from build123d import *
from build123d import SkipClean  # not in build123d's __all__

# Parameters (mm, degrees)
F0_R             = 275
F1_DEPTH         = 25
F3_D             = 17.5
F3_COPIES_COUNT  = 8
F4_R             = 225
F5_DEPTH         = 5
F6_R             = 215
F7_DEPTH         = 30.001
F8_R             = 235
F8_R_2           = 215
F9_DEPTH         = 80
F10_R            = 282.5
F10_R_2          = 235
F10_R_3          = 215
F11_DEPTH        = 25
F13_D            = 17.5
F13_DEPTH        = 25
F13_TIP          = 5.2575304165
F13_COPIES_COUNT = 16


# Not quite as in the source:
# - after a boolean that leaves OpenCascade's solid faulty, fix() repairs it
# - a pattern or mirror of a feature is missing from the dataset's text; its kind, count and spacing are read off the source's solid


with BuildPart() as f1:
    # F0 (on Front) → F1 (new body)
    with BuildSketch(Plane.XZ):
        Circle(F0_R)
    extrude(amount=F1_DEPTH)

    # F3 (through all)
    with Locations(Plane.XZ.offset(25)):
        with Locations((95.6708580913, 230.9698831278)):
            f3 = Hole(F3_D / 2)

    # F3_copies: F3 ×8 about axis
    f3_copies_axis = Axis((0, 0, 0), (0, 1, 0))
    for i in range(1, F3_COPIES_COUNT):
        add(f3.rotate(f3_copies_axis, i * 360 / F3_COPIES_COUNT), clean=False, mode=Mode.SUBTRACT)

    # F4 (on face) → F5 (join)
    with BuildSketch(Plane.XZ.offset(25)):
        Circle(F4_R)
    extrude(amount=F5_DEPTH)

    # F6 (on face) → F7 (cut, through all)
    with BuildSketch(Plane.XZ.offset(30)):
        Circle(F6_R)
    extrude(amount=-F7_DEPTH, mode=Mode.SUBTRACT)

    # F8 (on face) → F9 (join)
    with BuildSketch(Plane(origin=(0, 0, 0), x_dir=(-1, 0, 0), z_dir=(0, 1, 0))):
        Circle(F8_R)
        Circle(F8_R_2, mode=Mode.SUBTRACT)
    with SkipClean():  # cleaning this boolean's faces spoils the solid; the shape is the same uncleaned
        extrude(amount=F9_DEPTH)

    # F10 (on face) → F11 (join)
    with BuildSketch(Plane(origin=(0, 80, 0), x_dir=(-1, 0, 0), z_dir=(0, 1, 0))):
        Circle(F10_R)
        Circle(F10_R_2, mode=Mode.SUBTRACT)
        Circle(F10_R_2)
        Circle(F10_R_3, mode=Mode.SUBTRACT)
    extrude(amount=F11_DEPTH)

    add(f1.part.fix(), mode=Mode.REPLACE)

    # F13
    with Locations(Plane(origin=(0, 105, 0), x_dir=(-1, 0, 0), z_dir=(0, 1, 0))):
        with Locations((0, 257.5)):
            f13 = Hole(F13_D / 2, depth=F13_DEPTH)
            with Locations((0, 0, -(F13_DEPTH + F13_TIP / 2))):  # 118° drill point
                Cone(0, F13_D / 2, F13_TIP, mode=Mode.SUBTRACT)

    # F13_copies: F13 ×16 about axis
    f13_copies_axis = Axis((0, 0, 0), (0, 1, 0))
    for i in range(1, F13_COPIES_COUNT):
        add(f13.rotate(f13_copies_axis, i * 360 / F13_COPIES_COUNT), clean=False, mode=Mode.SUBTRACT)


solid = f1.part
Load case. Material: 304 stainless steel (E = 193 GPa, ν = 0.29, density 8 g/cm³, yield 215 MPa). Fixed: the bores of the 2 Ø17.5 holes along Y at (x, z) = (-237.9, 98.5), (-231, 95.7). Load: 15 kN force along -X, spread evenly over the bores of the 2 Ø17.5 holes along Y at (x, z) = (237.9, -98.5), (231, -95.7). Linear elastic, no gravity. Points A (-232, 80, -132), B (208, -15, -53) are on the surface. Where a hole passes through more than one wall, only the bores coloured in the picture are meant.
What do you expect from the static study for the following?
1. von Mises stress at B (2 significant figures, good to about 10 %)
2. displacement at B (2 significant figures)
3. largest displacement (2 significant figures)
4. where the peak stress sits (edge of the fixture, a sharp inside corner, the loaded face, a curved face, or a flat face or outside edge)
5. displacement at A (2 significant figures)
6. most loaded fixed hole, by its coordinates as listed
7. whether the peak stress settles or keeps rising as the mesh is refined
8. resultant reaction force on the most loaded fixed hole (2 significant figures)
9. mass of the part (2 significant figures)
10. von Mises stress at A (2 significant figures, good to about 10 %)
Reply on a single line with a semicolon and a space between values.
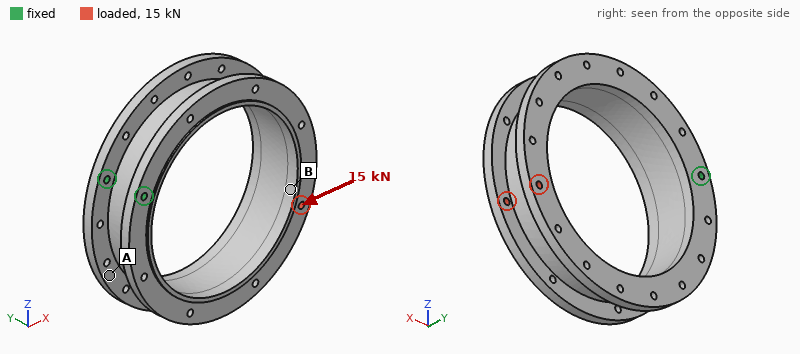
17 MPa; 0.65 mm; 0.74 mm; edge of the fixture; 0.32 mm; (-231, 95.7); keeps rising; 8.3 kN; 57 kg; 8.6 MPa
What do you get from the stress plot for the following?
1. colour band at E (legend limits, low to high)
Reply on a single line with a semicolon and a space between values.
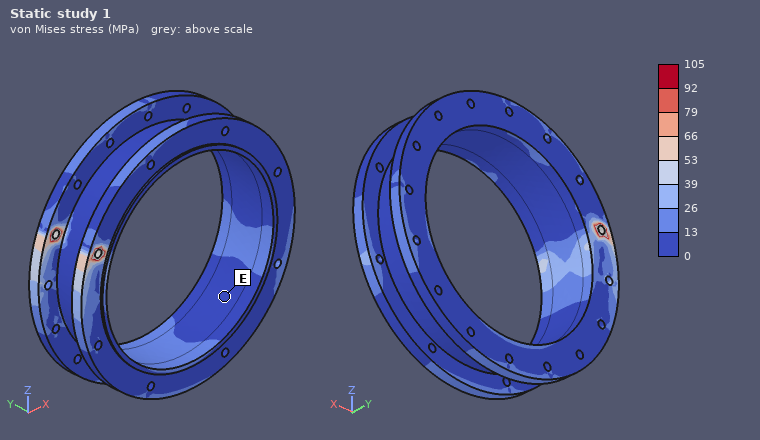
0 to 13 MPa
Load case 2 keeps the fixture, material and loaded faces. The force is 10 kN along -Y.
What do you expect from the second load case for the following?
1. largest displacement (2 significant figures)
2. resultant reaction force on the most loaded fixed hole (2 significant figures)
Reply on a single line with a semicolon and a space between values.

1.6 mm; 43 kN
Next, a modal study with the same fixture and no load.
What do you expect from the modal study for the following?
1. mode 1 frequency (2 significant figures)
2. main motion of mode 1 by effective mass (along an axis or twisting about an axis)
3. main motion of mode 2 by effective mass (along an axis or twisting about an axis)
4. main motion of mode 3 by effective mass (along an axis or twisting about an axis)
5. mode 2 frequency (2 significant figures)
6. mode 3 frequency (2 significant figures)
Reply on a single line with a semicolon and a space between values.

89 Hz; along Z; along Y; twisting about X; 110 Hz; 290 Hz
